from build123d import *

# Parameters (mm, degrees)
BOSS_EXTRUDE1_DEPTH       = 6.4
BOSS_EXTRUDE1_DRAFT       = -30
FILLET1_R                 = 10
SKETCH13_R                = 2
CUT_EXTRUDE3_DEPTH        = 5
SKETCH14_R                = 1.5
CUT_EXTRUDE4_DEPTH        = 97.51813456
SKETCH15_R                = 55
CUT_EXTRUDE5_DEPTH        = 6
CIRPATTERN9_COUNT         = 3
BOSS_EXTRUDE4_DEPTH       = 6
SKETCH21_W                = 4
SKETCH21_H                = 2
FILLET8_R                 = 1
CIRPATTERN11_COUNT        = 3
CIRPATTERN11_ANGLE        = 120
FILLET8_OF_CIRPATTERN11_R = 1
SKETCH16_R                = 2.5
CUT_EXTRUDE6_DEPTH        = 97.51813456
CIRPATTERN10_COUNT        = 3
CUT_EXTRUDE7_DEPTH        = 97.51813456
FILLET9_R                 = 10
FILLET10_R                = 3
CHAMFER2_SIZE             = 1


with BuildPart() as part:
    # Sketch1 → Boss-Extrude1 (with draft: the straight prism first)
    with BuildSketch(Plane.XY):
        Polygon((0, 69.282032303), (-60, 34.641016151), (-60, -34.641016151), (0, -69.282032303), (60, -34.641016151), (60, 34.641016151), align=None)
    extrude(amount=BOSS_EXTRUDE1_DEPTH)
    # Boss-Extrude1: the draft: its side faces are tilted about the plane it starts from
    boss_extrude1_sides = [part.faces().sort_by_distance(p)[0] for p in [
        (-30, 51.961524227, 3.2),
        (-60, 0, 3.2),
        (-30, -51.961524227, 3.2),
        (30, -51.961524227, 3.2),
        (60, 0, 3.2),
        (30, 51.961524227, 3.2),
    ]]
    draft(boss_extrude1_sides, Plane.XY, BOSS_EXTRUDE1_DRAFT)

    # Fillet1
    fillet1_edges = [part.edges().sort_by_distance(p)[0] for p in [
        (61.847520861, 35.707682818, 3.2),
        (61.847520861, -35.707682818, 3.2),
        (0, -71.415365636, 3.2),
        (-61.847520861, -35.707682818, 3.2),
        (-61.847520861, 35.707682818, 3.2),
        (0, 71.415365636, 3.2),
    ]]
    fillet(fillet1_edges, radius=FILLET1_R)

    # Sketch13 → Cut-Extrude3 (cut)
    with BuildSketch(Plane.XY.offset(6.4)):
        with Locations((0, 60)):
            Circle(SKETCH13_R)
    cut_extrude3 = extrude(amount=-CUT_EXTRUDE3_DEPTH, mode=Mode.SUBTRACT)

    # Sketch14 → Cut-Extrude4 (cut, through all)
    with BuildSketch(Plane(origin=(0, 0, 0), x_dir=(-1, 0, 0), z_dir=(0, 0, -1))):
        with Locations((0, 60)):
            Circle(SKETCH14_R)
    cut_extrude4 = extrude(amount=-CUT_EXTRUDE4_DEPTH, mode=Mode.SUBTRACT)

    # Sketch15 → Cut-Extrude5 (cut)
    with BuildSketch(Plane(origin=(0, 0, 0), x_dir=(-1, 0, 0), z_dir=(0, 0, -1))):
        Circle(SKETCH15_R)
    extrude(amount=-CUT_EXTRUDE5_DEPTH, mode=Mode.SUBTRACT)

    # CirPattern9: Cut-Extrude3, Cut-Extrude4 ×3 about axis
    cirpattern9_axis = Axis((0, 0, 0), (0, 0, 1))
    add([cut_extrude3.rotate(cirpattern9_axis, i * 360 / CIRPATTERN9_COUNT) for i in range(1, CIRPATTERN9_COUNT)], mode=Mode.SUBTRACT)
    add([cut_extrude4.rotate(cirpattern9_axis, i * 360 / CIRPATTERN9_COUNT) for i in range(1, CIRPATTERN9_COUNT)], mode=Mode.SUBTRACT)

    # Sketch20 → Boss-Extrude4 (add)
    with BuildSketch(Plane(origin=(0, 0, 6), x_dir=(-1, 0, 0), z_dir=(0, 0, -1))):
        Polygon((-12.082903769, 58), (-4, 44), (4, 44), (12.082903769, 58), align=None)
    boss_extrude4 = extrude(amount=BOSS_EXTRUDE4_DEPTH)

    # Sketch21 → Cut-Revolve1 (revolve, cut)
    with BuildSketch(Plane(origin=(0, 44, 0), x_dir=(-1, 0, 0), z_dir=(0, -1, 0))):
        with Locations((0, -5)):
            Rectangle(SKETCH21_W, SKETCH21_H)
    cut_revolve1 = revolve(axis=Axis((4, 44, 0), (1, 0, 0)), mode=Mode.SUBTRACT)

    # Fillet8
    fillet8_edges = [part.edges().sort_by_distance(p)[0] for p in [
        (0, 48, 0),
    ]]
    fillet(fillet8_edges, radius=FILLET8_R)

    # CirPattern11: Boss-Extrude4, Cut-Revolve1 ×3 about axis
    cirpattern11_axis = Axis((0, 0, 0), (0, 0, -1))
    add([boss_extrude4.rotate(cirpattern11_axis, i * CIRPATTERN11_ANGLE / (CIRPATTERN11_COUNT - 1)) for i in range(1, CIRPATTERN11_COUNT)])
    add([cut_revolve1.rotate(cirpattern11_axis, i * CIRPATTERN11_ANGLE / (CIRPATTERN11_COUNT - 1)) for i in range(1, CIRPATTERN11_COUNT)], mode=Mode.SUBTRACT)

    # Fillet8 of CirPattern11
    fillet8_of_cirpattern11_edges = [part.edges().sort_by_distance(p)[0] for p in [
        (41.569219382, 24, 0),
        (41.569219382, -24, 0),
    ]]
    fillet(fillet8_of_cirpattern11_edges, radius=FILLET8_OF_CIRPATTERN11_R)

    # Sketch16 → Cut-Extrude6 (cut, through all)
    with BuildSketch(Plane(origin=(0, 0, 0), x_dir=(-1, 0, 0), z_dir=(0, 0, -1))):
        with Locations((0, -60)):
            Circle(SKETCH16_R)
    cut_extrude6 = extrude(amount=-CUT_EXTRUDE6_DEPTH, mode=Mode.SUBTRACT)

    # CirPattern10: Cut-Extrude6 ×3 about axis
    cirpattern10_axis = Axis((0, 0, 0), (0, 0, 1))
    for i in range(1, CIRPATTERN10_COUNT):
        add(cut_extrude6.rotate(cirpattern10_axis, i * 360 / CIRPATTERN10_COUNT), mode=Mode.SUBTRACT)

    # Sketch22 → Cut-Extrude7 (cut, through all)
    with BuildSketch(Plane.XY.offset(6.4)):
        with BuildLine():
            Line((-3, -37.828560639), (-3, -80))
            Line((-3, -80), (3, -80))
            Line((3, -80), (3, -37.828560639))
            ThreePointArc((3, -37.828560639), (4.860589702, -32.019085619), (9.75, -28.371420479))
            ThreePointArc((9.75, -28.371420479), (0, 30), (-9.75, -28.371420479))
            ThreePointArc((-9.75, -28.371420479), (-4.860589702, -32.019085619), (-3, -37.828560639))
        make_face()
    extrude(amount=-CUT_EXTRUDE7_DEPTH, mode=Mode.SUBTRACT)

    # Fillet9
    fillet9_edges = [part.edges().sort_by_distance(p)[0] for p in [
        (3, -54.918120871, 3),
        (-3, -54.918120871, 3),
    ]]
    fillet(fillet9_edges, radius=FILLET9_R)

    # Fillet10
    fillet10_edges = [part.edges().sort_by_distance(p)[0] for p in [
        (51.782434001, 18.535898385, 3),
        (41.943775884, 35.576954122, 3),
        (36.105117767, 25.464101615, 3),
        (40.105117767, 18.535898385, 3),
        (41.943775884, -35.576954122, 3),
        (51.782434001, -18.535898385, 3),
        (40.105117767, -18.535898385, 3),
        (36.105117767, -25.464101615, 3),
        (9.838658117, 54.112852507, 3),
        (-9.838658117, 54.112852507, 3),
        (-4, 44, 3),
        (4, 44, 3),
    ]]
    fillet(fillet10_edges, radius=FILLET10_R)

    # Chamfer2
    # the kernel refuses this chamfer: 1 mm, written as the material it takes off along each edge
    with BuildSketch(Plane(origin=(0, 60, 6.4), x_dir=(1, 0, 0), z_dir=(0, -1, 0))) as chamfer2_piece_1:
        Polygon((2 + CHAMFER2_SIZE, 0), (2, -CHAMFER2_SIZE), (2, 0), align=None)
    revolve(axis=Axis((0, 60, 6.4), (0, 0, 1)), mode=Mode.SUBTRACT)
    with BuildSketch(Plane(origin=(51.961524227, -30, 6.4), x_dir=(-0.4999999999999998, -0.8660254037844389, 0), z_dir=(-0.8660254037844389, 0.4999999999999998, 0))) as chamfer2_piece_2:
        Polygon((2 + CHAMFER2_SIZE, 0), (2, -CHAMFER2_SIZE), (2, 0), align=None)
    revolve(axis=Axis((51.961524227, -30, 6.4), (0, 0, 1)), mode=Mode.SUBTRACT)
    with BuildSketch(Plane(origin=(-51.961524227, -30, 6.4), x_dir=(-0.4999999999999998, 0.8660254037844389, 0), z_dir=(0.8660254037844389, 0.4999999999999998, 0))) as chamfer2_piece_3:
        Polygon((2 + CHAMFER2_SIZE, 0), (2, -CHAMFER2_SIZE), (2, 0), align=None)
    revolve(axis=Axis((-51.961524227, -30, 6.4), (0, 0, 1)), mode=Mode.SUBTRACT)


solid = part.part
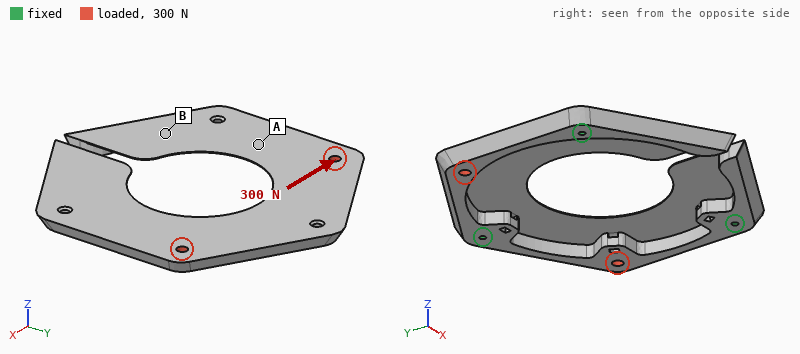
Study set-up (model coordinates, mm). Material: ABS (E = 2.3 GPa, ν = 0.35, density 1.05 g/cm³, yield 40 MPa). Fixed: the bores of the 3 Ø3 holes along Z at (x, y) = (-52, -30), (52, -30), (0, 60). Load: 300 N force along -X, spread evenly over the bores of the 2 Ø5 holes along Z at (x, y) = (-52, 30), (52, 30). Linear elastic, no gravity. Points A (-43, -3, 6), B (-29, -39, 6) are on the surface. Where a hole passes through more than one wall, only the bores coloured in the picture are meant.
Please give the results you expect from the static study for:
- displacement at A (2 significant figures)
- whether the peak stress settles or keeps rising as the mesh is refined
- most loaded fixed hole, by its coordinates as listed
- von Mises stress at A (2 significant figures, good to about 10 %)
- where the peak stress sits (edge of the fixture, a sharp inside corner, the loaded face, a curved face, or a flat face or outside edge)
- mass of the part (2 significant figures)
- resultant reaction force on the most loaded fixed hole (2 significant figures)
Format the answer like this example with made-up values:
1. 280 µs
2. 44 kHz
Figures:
1. 0.23 mm
2. keeps rising
3. (0, 60)
4. 3.2 MPa
5. edge of the fixture
6. 29 g
7. 250 N
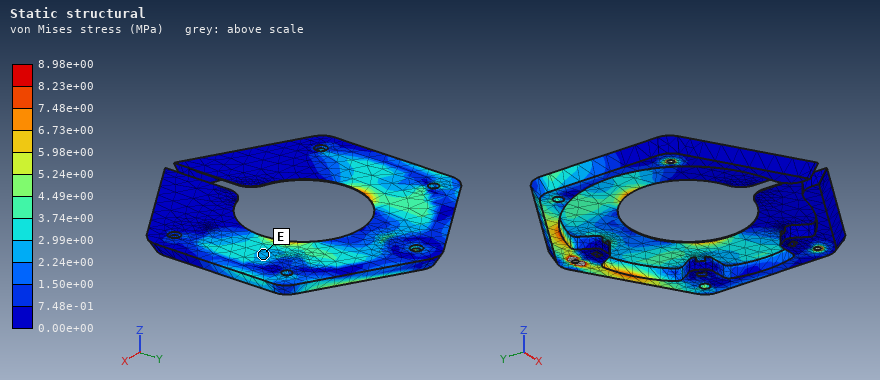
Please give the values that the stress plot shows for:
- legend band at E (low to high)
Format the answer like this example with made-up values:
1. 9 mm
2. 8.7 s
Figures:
1. 2.24e+00 to 2.99e+00 MPa
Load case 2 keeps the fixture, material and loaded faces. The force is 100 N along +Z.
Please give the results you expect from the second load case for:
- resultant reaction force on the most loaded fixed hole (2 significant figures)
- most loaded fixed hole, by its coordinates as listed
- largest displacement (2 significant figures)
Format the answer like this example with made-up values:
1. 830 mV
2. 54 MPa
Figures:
1. 110 N
2. (0, 60)
3. 2.1 mm
